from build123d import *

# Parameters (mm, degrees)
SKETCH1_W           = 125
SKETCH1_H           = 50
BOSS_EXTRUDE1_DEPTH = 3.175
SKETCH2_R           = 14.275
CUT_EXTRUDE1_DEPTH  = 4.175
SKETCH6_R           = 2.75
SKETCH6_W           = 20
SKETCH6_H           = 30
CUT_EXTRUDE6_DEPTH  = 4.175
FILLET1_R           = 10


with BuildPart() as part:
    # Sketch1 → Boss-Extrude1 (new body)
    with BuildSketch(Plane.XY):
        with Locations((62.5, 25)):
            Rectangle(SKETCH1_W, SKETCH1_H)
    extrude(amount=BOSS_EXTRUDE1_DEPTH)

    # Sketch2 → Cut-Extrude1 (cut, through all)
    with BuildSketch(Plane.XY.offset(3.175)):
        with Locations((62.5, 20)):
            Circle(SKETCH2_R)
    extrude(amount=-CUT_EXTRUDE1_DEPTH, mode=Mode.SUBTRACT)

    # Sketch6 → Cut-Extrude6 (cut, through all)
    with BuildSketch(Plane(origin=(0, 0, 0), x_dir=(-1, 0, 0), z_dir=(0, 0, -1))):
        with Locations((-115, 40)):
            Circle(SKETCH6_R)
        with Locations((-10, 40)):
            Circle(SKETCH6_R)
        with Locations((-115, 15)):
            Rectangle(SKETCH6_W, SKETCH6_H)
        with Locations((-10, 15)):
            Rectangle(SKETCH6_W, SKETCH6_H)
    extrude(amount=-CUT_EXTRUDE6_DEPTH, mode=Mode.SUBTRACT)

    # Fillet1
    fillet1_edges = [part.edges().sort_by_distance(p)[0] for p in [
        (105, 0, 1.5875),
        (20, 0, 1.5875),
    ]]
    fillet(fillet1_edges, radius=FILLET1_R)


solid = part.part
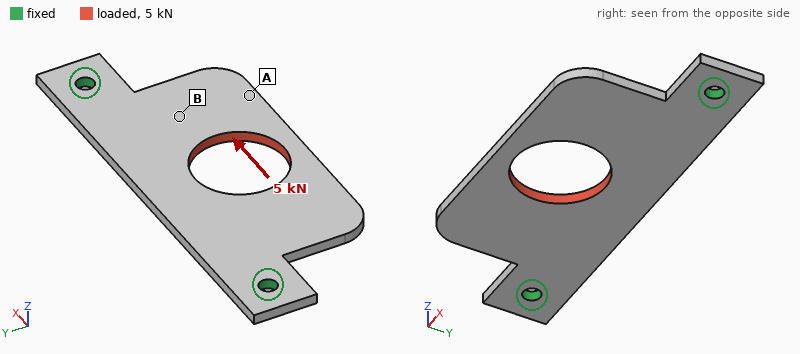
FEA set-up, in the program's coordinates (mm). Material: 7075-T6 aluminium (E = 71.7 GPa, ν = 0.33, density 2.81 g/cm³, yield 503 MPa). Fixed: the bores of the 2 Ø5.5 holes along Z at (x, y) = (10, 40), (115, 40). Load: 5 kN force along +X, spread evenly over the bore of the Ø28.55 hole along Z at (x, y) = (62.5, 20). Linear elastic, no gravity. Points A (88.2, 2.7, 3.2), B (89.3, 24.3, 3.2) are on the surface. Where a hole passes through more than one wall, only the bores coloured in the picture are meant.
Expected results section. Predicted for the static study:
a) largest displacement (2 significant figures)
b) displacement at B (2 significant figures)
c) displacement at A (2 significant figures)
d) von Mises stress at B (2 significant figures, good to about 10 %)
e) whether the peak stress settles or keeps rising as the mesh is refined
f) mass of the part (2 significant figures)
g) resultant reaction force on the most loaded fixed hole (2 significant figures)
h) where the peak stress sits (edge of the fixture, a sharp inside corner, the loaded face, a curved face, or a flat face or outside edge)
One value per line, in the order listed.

59 µm
25 µm
52 µm
34 MPa
keeps rising
39 g
2.7 kN
a sharp inside corner
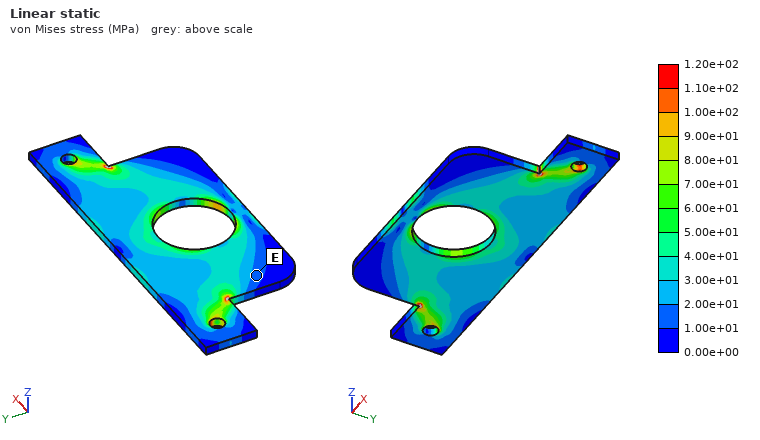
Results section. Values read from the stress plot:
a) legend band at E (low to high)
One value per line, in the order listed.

1.00e+01 to 2.00e+01 MPa
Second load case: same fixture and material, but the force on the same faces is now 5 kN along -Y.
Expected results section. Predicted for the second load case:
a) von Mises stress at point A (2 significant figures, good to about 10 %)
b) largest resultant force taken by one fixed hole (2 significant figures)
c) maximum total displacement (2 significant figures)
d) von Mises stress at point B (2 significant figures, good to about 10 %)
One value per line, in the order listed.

31 MPa
2.8 kN
0.11 mm
45 MPa
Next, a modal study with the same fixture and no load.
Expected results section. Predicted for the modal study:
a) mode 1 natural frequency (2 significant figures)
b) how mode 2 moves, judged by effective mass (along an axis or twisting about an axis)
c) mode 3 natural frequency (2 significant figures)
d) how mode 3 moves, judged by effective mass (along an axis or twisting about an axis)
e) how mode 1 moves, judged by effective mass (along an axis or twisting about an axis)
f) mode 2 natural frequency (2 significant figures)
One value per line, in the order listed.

860 Hz
along Z
2000 Hz
twisting about Y
along Z
1700 Hz
